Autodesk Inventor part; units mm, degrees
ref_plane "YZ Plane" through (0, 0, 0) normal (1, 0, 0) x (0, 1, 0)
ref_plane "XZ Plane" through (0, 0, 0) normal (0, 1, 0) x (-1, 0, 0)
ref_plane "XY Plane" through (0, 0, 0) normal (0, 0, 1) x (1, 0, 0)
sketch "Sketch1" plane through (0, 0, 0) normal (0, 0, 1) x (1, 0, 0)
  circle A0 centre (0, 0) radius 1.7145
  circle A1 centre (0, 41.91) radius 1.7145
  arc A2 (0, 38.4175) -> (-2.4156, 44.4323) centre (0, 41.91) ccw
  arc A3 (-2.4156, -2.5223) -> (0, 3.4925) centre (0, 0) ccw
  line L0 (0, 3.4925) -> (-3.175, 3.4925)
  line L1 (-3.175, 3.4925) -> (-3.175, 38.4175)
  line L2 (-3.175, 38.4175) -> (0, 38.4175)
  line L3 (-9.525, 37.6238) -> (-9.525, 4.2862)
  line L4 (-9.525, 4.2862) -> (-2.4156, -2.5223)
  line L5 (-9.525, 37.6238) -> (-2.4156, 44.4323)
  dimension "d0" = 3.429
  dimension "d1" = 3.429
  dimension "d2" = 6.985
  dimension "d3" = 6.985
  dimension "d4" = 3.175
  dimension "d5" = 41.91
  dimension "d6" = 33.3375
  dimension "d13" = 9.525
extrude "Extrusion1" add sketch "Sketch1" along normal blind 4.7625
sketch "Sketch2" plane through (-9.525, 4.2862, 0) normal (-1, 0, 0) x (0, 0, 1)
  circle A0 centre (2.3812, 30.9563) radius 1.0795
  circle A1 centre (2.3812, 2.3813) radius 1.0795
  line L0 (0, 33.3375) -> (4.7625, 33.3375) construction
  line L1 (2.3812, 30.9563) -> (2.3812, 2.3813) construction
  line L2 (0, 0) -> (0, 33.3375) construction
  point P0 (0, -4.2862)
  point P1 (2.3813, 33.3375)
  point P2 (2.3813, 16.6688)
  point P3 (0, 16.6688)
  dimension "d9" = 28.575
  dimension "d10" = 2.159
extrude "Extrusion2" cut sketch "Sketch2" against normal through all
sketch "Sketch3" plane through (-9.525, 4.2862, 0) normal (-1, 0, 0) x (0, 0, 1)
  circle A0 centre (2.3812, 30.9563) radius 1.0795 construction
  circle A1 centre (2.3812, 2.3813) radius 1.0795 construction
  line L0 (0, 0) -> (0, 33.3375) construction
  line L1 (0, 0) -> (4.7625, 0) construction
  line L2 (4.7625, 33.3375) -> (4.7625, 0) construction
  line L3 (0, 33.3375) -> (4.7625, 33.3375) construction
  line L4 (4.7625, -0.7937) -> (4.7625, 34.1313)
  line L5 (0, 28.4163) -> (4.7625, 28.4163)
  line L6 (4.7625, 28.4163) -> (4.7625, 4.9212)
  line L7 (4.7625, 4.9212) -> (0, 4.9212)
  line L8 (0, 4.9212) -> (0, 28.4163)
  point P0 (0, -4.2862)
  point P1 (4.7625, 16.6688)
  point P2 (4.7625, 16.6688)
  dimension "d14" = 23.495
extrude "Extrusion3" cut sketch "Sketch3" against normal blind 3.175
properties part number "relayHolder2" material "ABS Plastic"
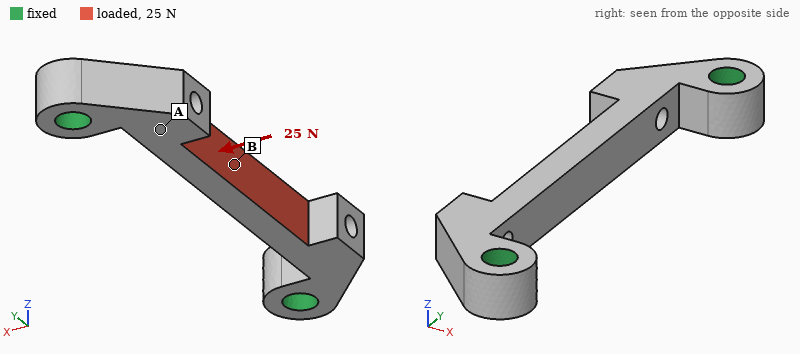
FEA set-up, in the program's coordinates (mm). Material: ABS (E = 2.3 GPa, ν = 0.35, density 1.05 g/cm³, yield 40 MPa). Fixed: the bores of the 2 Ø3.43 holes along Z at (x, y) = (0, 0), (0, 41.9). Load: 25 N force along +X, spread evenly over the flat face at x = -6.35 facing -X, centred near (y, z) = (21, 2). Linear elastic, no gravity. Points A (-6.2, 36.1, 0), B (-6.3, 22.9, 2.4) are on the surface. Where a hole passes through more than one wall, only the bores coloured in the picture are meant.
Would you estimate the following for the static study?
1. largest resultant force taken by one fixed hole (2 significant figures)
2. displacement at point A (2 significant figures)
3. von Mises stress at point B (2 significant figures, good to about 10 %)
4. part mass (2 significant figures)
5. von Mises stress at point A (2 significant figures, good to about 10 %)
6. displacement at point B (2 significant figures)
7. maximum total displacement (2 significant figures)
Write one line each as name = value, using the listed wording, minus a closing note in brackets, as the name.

largest resultant force taken by one fixed hole = 16 N
displacement at point A = 0.036 mm
von Mises stress at point B = 6.9 MPa
part mass = 1.1 g
von Mises stress at point A = 2.0 MPa
displacement at point B = 0.17 mm
maximum total displacement = 0.17 mm
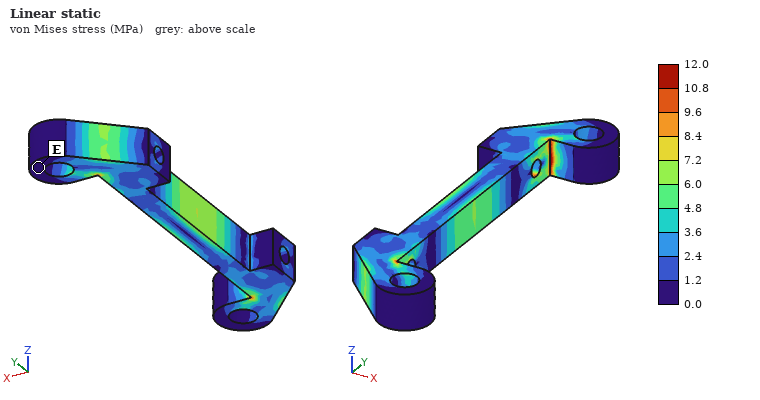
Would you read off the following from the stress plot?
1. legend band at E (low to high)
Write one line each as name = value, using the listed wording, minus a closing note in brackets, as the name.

legend band at E = 0.0 to 1.2 MPa
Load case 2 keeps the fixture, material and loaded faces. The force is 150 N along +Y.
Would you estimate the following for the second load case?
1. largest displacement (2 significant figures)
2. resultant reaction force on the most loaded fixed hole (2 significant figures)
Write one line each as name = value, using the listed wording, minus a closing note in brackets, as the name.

largest displacement = 54 µm
resultant reaction force on the most loaded fixed hole = 76 N
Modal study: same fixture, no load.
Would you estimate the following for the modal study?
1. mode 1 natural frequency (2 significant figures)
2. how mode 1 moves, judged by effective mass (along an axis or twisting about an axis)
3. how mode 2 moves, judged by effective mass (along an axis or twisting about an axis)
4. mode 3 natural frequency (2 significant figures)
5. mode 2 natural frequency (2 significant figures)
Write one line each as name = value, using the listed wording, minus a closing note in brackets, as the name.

mode 1 natural frequency = 3300 Hz
how mode 1 moves, judged by effective mass = along X
how mode 2 moves, judged by effective mass = along Z
mode 3 natural frequency = 6700 Hz
mode 2 natural frequency = 3500 Hz
